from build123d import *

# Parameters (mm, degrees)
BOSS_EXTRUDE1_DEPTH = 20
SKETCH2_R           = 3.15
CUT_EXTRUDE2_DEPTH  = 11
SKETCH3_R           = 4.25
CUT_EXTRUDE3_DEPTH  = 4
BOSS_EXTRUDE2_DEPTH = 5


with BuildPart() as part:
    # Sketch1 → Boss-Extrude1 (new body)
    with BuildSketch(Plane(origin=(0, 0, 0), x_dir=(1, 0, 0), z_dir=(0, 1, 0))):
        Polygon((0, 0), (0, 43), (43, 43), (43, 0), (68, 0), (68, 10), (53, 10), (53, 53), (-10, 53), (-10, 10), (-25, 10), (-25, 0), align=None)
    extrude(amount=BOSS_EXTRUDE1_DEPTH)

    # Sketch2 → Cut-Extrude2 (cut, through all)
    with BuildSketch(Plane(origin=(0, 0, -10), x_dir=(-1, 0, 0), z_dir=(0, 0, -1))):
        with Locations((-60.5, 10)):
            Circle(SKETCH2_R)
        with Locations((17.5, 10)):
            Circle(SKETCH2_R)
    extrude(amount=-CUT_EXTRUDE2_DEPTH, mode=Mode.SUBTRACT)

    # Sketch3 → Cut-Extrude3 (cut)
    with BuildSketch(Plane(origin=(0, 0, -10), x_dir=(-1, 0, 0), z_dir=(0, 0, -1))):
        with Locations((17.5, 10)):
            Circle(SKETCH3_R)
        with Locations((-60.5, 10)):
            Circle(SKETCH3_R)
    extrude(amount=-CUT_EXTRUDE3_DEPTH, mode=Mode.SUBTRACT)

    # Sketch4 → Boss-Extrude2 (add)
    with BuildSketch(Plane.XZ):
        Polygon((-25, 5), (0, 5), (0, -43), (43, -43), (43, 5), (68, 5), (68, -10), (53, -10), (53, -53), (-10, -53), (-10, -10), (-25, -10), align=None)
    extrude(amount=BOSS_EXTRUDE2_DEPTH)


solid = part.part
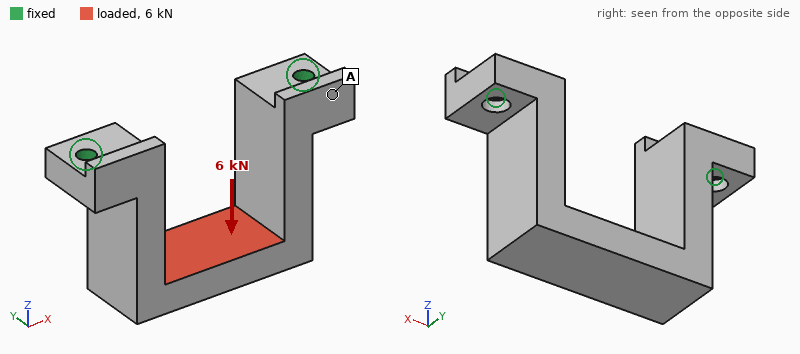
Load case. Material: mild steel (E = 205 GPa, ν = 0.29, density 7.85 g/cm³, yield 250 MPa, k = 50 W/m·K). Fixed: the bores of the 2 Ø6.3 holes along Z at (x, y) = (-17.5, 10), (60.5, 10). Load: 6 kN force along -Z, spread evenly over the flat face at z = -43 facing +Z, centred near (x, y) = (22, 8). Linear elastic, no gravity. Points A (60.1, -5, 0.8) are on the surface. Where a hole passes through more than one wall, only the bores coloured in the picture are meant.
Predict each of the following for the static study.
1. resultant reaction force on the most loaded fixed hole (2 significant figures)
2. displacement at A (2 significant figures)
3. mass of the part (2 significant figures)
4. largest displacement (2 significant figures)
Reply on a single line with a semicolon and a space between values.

3.2 kN; 5.0 µm; 350 g; 25 µm
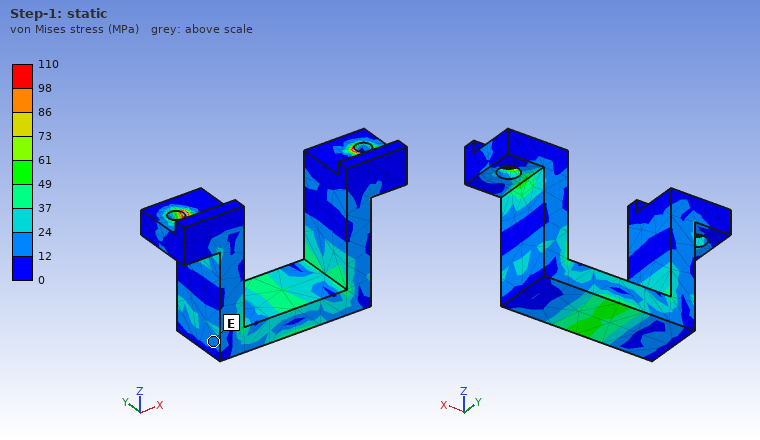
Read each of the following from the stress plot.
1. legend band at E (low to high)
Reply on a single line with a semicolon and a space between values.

12 to 24 MPa
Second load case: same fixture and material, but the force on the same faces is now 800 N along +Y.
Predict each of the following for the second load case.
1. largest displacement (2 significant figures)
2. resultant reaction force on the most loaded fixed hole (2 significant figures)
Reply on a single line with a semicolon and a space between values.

33 µm; 400 N
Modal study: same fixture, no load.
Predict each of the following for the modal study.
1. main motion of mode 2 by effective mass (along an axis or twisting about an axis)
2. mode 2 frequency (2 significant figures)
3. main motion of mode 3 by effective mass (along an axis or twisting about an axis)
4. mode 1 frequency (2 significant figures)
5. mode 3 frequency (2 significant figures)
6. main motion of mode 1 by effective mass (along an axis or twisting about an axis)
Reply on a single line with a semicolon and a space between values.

along X; 3100 Hz; twisting about Z; 1900 Hz; 4200 Hz; along Y
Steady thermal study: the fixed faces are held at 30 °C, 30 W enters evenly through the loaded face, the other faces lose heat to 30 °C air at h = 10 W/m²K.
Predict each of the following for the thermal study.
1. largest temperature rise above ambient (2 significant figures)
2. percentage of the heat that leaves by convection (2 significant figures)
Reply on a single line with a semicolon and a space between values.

72 K; 13 %
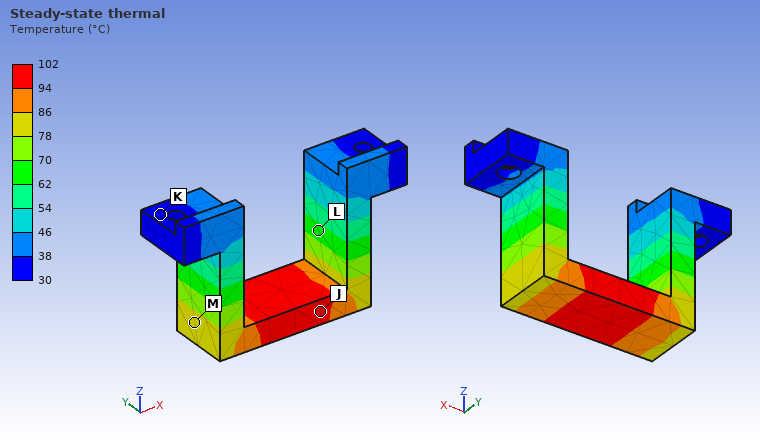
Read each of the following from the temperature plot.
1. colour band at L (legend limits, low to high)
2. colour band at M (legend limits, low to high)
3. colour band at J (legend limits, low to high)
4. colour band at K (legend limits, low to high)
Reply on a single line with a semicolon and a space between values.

62 to 70 °C; 78 to 86 °C; 94 to 102 °C; 30 to 38 °C
